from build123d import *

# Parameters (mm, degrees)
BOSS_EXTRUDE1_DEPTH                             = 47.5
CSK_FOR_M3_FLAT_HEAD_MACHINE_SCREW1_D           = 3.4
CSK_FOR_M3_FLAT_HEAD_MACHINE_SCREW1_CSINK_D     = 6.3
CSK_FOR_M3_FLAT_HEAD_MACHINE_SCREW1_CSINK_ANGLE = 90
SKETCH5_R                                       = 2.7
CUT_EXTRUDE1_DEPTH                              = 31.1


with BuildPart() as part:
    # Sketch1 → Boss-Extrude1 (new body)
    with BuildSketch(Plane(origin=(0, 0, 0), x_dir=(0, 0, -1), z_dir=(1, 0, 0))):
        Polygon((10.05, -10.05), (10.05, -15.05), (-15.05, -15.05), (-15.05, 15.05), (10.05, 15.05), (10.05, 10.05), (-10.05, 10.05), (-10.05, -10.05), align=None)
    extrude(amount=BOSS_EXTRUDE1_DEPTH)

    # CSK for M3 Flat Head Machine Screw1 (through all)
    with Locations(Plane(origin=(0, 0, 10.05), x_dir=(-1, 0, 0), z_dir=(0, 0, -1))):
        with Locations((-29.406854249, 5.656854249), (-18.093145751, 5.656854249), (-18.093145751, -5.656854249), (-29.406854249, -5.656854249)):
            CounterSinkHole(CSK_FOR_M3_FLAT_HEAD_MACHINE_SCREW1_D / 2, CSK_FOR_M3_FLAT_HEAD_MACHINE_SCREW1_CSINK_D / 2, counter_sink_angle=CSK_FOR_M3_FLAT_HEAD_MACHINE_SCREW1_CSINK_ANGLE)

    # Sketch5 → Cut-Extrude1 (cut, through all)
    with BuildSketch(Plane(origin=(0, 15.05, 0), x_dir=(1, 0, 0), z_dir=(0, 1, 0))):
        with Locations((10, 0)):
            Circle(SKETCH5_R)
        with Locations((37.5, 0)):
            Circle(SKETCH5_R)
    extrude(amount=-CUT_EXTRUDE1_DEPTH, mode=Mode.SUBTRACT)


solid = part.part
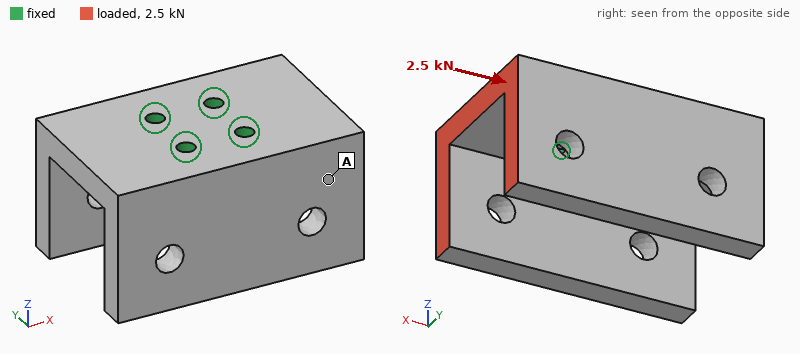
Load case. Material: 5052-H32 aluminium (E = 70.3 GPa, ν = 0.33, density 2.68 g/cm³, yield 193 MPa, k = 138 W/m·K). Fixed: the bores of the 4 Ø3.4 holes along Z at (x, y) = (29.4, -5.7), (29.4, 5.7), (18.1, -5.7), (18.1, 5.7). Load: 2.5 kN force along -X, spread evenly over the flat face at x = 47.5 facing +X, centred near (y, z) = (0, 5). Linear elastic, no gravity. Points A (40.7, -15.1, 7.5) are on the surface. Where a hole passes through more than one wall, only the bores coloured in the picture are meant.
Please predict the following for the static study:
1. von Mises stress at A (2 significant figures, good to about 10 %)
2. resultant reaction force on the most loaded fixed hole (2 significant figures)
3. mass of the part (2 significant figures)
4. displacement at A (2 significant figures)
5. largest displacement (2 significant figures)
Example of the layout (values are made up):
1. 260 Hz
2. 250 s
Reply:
1. 8.0 MPa
2. 1.0 kN
3. 43 g
4. 17 µm
5. 33 µm
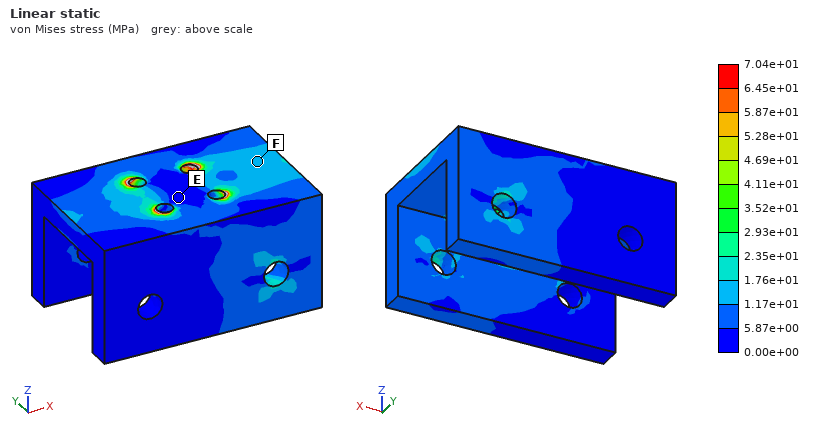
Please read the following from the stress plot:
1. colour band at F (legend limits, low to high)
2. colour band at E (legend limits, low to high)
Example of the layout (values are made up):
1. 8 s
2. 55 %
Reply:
1. 1.17e+01 to 1.76e+01 MPa
2. 0.00e+00 to 5.87e+00 MPa
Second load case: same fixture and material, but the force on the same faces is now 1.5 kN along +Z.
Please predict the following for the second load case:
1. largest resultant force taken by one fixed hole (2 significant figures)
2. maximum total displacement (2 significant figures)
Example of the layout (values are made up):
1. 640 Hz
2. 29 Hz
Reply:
1. 1.5 kN
2. 65 µm
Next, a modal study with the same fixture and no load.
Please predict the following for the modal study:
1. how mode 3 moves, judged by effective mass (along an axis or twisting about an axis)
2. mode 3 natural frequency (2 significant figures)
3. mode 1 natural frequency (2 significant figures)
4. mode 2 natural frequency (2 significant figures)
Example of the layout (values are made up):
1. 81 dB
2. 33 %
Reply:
1. along X
2. 6600 Hz
3. 5100 Hz
4. 5200 Hz
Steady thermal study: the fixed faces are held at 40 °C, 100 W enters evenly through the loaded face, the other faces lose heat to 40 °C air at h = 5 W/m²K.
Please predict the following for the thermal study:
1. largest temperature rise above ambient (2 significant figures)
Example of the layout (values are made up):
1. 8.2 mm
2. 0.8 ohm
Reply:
1. 64 K
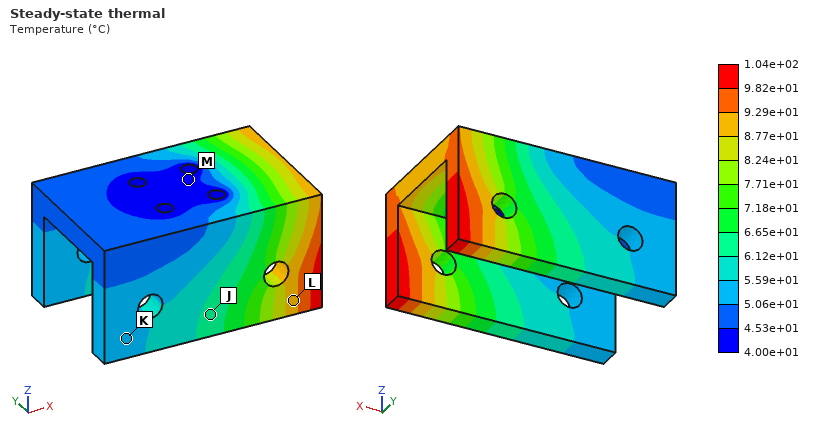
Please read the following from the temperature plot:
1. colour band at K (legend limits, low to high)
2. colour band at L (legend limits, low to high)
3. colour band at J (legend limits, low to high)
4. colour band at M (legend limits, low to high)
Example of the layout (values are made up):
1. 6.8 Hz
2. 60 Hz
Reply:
1. 5.06e+01 to 5.59e+01 °C
2. 8.77e+01 to 9.29e+01 °C
3. 6.12e+01 to 6.65e+01 °C
4. 4.00e+01 to 4.53e+01 °C
